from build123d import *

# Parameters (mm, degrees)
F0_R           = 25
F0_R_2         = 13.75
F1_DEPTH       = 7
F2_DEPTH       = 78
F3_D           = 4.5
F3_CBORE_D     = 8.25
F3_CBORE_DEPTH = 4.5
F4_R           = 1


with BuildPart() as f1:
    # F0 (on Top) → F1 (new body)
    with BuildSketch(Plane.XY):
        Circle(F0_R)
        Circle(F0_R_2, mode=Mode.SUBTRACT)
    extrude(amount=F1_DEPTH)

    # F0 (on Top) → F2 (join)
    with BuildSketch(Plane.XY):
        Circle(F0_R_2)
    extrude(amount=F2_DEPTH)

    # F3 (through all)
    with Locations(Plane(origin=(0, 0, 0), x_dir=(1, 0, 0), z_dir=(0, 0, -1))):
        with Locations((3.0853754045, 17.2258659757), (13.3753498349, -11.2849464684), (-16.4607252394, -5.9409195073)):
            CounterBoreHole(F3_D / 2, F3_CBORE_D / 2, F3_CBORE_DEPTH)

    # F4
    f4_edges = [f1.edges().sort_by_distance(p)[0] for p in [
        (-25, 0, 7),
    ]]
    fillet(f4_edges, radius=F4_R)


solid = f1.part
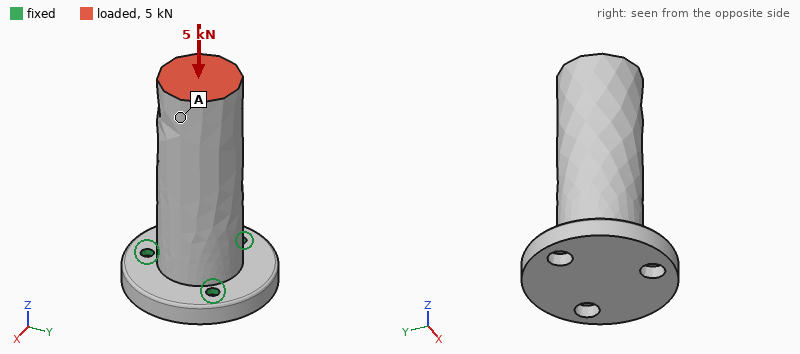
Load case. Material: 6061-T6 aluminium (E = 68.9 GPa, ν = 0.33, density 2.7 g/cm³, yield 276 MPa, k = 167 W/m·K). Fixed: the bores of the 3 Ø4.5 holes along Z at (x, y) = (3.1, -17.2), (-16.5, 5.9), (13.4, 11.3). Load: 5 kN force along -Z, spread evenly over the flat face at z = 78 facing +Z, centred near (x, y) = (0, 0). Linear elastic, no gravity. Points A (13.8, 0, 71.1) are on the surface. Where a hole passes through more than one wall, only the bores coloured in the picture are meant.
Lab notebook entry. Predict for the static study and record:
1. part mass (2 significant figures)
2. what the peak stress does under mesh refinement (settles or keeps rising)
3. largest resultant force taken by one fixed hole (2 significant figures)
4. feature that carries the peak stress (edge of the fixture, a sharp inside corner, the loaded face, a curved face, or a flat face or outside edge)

150 g
keeps rising
1.7 kN
edge of the fixture
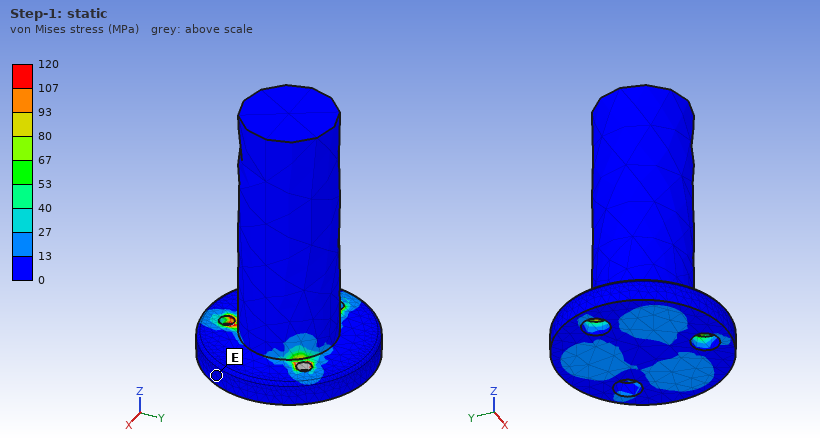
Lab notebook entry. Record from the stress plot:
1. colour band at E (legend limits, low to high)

0 to 13 MPa
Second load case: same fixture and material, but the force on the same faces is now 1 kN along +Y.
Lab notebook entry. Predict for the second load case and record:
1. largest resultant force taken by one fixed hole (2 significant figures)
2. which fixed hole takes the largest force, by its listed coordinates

2.7 kN
(3.1, -17.2)
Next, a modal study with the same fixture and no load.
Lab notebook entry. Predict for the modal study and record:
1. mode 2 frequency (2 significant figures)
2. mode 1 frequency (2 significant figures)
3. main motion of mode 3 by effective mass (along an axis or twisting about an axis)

2200 Hz
2200 Hz
along Z
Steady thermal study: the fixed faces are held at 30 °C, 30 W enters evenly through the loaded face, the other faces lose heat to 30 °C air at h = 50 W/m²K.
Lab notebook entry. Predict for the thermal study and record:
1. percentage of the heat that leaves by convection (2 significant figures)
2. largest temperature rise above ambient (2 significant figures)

17 %
24 K
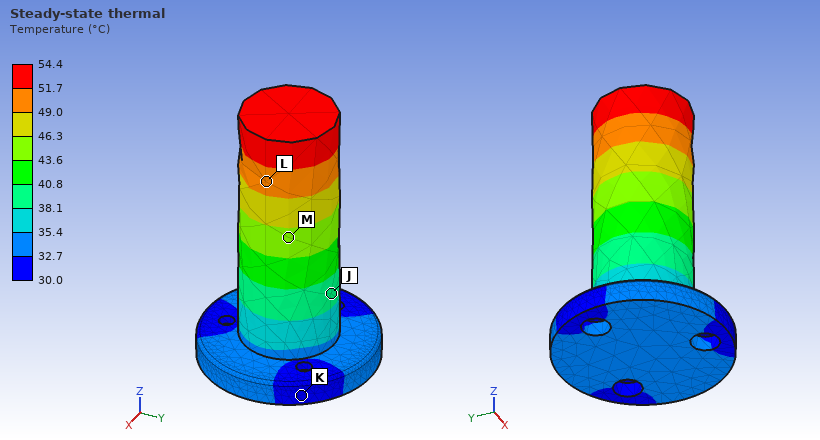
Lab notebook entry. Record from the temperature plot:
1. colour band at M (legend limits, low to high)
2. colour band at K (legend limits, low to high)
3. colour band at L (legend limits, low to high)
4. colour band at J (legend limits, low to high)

43.6 to 46.3 °C
30.0 to 32.7 °C
49.0 to 51.7 °C
38.1 to 40.8 °C
